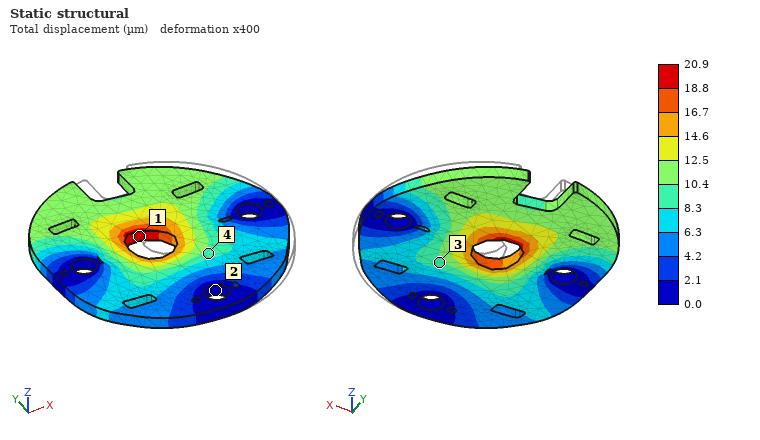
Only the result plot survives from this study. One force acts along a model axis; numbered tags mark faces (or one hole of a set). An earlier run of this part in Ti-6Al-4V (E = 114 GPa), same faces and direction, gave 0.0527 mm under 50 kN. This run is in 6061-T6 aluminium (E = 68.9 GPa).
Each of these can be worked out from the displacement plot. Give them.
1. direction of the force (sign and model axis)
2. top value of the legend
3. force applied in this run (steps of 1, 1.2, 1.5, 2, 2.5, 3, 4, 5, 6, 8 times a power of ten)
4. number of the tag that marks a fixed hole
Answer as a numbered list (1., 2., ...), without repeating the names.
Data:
1. -X
2. 20.9 µm
3. 12 kN
4. 2
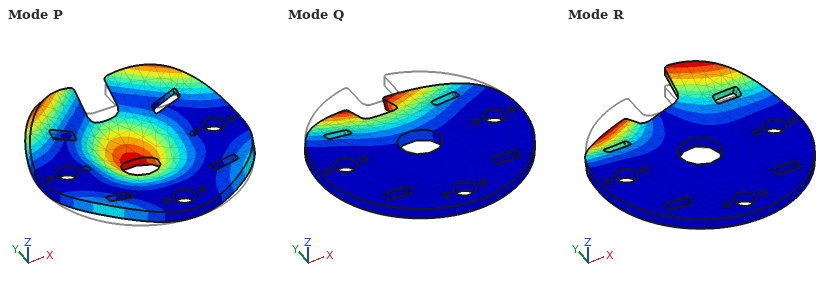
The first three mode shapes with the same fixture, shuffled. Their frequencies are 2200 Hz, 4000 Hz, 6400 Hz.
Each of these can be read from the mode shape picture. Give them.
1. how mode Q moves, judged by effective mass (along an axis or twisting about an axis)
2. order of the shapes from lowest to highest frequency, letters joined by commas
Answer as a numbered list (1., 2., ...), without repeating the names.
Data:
1. along Z
2. Q, R, P
